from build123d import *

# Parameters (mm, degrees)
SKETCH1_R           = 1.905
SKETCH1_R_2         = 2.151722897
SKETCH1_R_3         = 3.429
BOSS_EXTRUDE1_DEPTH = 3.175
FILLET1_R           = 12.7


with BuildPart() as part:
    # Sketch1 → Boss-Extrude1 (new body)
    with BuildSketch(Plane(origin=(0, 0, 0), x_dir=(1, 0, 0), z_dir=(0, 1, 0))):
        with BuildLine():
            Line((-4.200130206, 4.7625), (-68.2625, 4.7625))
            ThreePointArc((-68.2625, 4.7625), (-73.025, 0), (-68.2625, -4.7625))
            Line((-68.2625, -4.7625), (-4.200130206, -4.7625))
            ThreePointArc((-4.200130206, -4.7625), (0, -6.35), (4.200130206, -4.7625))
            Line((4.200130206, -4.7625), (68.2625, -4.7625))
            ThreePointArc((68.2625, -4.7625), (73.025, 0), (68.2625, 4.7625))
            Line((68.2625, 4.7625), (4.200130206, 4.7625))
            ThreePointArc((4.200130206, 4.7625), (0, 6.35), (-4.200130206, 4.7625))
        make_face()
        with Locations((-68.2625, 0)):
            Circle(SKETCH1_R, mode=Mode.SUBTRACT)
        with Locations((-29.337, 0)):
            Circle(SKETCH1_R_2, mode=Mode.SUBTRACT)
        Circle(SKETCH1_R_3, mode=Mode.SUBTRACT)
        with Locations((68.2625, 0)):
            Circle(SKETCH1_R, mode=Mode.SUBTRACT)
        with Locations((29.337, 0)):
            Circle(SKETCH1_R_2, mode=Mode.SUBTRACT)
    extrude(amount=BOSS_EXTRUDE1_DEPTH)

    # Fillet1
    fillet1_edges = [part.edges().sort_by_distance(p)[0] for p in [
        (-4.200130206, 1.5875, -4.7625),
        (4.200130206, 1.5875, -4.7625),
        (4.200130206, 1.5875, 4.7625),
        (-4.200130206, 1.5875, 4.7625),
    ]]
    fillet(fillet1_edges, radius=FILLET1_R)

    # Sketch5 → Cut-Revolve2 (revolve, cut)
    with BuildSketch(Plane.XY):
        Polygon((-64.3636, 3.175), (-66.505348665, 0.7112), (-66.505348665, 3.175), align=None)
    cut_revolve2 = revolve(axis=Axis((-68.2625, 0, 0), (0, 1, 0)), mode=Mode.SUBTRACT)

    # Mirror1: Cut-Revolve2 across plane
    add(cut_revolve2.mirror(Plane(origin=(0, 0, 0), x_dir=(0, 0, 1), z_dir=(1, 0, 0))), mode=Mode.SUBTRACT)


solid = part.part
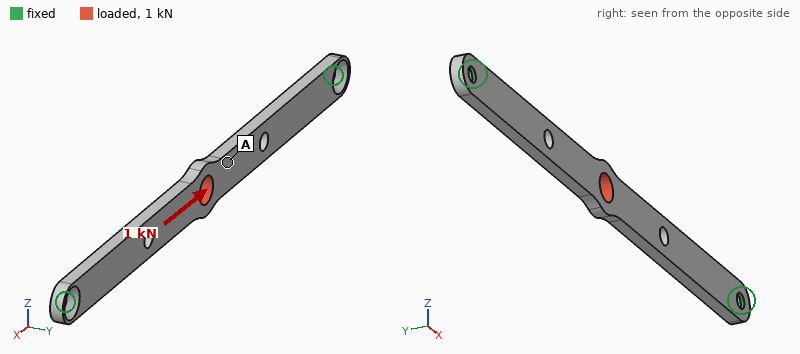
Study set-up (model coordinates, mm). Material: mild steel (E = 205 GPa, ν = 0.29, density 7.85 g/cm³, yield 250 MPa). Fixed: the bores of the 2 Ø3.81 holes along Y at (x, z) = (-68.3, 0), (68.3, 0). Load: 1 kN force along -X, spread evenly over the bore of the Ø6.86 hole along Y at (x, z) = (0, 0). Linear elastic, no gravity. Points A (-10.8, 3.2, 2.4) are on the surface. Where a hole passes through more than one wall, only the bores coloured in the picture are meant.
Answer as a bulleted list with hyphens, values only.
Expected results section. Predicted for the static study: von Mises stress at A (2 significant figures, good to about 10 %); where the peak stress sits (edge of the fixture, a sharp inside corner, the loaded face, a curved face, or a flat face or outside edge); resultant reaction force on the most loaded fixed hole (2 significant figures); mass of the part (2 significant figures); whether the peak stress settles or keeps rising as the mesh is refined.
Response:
- 15 MPa
- edge of the fixture
- 500 N
- 32 g
- keeps rising
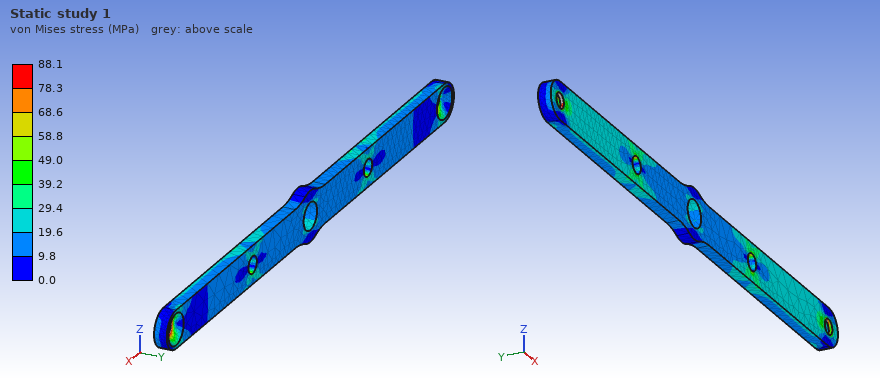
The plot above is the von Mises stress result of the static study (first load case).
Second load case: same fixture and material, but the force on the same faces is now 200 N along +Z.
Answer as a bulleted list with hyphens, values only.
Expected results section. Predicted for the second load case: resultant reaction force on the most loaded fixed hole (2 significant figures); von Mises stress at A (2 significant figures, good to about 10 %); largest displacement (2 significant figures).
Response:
- 100 N
- 30 MPa
- 76 µm
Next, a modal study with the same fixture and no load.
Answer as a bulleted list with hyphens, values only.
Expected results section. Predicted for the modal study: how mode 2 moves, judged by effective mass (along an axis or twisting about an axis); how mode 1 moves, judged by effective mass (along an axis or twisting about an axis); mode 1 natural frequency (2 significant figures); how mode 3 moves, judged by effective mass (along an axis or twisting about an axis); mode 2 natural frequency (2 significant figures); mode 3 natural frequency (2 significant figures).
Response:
- twisting about Z
- along Y
- 790 Hz
- along Z
- 2200 Hz
- 2300 Hz
